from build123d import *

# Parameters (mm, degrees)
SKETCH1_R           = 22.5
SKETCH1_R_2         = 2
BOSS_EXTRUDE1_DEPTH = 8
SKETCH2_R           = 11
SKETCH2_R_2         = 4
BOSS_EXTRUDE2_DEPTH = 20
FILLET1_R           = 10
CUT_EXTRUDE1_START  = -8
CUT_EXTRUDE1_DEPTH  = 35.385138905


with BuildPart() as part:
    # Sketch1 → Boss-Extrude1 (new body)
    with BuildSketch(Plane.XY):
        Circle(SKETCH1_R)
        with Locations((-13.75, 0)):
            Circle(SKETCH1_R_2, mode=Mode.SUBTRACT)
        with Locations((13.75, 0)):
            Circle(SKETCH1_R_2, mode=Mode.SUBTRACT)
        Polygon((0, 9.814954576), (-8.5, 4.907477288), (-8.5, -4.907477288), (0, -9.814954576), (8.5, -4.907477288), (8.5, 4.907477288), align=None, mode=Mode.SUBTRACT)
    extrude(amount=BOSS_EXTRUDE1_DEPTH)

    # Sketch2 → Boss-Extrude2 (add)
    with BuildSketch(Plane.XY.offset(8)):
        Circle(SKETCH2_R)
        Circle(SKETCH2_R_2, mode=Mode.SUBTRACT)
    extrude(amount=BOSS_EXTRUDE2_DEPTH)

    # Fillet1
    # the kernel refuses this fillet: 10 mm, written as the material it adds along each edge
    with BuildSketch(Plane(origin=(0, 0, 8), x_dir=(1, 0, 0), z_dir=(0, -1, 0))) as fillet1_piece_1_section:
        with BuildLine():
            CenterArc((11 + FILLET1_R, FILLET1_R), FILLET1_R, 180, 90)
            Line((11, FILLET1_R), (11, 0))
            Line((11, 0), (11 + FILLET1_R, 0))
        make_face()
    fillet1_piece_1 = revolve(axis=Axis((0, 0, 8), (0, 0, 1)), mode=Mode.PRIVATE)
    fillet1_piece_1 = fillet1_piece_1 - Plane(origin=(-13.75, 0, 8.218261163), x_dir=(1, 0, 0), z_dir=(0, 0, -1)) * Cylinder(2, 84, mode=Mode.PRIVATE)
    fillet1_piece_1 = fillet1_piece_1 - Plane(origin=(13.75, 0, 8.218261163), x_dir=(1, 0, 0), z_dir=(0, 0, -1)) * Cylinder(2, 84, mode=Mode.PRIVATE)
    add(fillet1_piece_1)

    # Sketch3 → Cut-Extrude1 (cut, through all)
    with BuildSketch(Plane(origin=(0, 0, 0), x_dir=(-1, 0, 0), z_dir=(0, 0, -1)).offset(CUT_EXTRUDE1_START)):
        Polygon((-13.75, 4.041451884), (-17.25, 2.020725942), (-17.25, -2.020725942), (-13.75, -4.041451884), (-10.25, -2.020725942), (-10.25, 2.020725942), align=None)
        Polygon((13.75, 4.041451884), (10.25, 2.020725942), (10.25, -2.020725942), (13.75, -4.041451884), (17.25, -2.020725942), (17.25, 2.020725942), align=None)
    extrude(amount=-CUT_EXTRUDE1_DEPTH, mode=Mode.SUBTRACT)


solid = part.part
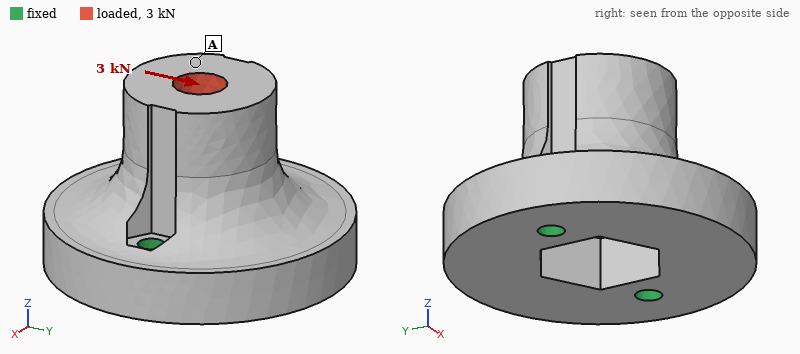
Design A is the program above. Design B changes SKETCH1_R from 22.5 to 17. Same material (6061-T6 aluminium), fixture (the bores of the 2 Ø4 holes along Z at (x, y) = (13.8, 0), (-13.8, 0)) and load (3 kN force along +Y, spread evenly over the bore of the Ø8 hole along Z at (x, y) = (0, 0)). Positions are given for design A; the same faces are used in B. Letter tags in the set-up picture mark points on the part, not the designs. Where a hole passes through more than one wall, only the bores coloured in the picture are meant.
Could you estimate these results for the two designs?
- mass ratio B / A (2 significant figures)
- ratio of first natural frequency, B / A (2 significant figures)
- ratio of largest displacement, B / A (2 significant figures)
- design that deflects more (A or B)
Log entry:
0.71
1.1
1.2
B
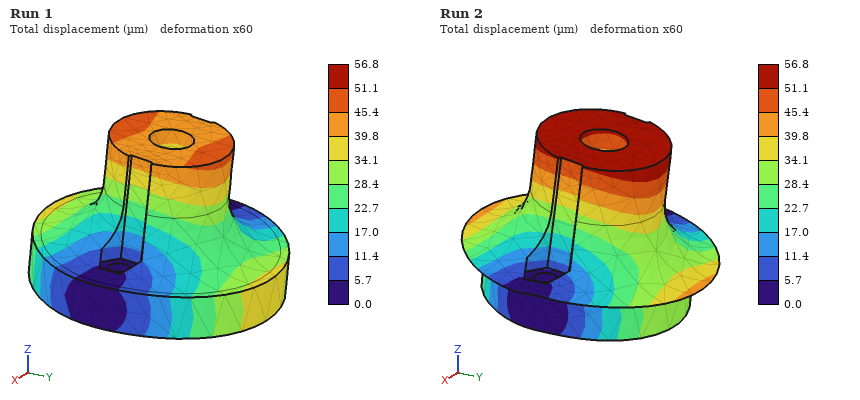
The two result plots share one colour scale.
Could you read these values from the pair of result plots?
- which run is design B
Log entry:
Run 2
